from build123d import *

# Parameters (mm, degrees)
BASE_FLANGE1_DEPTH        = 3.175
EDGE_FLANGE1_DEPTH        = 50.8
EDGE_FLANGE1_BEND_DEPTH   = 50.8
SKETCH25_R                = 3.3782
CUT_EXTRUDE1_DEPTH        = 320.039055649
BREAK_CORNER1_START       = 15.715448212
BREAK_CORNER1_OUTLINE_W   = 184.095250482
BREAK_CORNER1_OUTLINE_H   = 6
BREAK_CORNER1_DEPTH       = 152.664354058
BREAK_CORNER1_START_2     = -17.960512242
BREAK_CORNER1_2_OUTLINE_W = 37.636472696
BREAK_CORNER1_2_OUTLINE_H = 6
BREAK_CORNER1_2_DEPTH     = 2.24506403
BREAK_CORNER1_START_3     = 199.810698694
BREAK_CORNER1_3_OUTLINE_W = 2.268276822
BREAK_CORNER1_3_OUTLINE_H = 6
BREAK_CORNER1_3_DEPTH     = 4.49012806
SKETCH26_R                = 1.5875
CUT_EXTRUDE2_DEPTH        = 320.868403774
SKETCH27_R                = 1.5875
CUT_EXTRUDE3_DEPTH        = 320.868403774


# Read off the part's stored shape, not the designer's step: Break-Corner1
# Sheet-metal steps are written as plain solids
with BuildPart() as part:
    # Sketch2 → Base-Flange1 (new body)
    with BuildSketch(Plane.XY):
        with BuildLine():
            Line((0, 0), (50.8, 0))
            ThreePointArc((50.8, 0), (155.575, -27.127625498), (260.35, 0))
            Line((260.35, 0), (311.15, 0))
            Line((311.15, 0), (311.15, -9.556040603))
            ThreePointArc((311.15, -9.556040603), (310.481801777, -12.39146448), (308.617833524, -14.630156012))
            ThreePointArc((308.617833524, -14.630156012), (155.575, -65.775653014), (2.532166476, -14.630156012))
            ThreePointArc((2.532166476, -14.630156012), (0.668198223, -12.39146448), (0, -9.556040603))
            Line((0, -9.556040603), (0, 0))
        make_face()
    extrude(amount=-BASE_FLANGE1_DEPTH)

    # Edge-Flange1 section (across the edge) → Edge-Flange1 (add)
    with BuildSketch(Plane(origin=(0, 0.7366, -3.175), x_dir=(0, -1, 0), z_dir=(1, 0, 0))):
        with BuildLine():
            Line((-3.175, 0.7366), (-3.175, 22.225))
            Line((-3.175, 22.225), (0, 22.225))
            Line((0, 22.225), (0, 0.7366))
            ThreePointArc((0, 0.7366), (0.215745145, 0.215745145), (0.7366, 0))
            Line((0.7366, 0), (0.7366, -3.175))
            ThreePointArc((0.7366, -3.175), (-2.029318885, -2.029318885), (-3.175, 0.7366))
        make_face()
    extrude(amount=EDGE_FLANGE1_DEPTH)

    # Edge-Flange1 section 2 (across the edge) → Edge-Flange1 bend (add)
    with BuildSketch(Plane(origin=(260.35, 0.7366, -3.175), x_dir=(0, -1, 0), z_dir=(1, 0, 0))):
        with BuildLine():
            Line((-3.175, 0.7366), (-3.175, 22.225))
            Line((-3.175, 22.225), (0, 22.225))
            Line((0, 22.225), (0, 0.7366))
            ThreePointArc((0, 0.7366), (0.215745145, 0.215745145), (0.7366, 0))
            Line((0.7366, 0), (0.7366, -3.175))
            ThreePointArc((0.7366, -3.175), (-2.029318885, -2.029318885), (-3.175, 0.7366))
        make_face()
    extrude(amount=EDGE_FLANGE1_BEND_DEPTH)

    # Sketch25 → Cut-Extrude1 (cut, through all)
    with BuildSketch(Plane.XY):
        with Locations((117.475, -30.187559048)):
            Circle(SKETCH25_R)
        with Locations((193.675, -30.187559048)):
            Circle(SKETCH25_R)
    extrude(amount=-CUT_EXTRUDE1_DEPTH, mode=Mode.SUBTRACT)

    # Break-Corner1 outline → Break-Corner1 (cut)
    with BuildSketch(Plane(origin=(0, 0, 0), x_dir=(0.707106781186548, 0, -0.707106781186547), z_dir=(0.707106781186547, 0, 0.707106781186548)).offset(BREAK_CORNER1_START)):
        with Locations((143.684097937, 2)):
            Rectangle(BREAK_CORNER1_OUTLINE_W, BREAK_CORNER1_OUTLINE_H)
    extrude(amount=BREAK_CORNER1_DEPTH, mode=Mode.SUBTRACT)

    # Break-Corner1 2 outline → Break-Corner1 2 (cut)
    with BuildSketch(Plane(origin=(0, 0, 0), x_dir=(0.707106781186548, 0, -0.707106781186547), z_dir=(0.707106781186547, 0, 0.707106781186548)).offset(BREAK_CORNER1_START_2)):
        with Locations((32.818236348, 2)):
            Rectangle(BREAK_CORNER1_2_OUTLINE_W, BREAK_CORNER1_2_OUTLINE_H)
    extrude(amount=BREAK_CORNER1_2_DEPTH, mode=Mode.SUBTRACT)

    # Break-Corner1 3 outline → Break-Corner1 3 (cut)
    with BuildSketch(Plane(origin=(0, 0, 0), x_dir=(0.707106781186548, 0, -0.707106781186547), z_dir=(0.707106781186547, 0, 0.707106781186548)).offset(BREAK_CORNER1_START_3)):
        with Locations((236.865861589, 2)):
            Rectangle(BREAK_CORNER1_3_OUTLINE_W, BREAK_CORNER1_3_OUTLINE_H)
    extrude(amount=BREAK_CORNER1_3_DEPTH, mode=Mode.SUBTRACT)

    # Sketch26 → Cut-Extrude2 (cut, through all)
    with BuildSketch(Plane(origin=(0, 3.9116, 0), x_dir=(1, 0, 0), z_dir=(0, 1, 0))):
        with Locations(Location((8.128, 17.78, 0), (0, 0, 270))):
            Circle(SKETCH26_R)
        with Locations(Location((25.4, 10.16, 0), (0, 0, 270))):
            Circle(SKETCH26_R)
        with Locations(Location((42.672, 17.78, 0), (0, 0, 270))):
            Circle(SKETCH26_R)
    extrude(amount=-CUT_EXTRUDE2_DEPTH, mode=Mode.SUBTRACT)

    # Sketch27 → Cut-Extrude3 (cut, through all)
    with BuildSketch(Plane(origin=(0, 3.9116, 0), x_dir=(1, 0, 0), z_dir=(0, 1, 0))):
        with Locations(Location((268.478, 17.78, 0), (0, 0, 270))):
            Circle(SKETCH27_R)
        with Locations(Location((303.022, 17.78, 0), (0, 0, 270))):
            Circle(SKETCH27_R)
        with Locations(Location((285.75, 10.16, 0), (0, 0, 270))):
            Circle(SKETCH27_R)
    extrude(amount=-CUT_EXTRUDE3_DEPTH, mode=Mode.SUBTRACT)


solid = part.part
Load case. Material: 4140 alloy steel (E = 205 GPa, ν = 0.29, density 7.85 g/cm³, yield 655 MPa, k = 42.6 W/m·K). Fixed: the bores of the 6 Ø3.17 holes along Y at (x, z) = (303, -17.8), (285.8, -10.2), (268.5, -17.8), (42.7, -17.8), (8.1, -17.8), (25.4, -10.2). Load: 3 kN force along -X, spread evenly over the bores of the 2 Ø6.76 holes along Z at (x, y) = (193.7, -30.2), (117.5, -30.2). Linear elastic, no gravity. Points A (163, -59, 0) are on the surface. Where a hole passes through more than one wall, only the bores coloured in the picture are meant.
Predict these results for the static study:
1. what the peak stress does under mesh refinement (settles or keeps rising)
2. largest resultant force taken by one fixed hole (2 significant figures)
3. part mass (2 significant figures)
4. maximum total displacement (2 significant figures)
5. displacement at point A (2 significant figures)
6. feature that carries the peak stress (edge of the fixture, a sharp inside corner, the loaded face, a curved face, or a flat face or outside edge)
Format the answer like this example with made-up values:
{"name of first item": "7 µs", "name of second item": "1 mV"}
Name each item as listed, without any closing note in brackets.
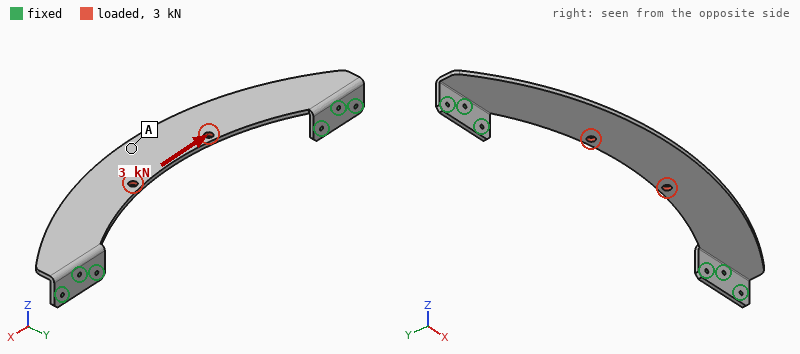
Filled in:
{"what the peak stress does under mesh refinement": "keeps rising", "largest resultant force taken by one fixed hole": "1.1 kN", "part mass": "340 g", "maximum total displacement": "32 µm", "displacement at point A": "19 µm", "feature that carries the peak stress": "edge of the fixture"}
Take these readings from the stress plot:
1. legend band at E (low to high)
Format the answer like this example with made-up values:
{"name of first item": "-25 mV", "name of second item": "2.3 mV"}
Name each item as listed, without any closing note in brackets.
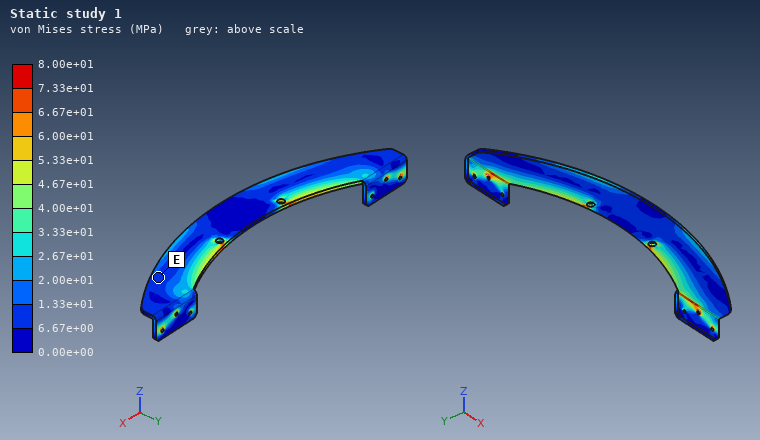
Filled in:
{"legend band at E": "6.67e+00 to 1.33e+01 MPa"}
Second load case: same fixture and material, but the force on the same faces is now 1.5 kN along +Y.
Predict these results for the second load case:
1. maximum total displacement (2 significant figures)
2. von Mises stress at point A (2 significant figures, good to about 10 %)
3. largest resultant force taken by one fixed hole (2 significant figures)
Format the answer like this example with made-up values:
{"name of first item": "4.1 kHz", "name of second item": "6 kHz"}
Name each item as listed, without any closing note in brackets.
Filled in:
{"maximum total displacement": "0.12 mm", "von Mises stress at point A": "19 MPa", "largest resultant force taken by one fixed hole": "1.1 kN"}
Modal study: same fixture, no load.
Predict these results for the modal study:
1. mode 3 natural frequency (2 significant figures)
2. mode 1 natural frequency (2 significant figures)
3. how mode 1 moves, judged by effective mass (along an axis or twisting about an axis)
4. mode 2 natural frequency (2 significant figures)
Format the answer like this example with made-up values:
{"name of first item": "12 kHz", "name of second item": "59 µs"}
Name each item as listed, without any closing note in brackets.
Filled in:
{"mode 3 natural frequency": "900 Hz", "mode 1 natural frequency": "210 Hz", "how mode 1 moves, judged by effective mass": "along Z", "mode 2 natural frequency": "570 Hz"}
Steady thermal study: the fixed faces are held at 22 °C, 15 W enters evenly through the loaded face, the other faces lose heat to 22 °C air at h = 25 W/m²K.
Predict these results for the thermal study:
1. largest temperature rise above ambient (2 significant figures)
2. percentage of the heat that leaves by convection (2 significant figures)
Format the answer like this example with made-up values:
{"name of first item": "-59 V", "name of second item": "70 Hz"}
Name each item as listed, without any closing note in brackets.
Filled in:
{"largest temperature rise above ambient": "59 K", "percentage of the heat that leaves by convection": "86 %"}
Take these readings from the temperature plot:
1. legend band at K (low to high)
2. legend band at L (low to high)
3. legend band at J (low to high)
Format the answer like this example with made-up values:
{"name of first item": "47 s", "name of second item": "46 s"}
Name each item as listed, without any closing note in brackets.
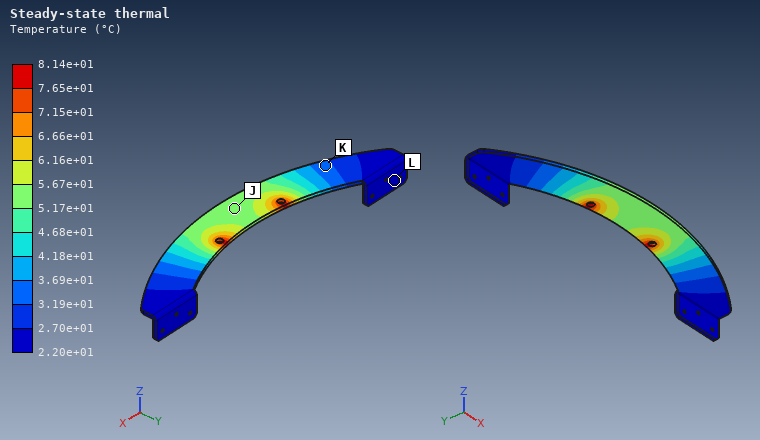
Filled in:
{"legend band at K": "3.19e+01 to 3.69e+01 °C", "legend band at L": "2.20e+01 to 2.70e+01 °C", "legend band at J": "5.17e+01 to 5.67e+01 °C"}
